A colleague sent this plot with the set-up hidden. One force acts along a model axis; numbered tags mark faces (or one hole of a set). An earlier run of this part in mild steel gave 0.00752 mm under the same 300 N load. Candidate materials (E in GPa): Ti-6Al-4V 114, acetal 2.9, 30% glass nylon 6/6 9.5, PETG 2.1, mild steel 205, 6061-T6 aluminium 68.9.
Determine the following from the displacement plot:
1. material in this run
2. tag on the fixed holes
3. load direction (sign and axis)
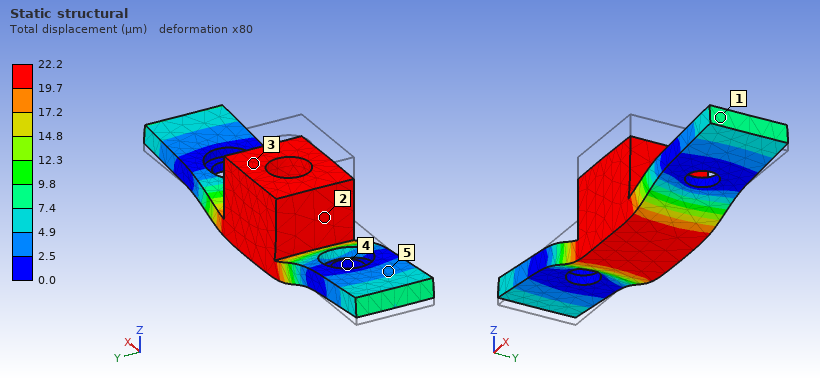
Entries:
6061-T6 aluminium
4
-Z
